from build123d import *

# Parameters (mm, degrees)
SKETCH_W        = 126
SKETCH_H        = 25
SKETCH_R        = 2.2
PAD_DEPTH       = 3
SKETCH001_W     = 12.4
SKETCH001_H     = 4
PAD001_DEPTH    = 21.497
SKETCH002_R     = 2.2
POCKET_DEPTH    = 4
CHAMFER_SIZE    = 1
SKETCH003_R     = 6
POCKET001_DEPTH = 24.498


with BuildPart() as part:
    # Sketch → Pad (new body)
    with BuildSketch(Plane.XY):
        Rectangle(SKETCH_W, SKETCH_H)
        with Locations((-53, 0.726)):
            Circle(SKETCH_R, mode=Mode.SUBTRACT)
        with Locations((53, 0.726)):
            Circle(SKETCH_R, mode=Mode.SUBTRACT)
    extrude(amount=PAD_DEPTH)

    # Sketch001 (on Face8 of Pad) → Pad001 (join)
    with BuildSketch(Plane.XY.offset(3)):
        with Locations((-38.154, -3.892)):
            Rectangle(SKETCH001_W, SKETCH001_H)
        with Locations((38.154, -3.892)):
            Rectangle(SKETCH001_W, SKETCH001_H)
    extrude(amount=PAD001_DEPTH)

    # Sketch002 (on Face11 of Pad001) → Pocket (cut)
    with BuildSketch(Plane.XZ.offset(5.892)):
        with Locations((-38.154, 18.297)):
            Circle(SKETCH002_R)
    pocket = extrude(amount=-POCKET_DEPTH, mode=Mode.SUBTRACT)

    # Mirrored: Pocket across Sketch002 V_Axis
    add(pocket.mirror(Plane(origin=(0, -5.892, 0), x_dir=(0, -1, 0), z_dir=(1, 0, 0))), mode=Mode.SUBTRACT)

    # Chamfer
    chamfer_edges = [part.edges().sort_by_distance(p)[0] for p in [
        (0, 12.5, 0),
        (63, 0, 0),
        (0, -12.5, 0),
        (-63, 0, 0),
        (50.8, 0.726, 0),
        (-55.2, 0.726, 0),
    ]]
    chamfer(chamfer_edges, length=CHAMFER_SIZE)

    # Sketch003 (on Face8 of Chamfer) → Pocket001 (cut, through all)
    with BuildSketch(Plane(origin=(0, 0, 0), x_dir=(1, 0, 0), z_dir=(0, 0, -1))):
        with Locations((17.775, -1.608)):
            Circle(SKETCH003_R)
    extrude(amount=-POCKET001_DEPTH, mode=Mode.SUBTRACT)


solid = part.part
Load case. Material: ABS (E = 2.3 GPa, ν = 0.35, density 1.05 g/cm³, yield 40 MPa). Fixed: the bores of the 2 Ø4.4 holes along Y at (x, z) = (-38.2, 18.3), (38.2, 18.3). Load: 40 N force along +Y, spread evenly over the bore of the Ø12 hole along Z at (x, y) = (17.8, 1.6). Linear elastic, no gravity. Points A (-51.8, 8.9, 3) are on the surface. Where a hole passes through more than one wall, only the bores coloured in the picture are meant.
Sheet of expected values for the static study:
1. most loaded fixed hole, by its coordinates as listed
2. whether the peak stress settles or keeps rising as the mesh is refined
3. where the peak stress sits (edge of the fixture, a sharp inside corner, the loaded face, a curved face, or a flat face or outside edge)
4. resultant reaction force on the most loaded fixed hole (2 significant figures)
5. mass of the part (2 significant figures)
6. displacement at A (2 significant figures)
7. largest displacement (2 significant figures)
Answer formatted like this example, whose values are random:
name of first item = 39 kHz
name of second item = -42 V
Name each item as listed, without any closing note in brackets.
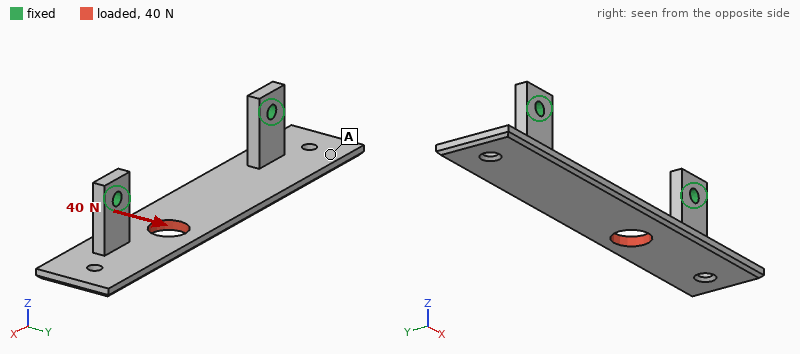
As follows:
most loaded fixed hole, by its coordinates as listed = (38.2, 18.3)
whether the peak stress settles or keeps rising as the mesh is refined = keeps rising
where the peak stress sits = edge of the fixture
resultant reaction force on the most loaded fixed hole = 29 N
mass of the part = 11 g
displacement at A = 0.15 mm
largest displacement = 0.42 mm
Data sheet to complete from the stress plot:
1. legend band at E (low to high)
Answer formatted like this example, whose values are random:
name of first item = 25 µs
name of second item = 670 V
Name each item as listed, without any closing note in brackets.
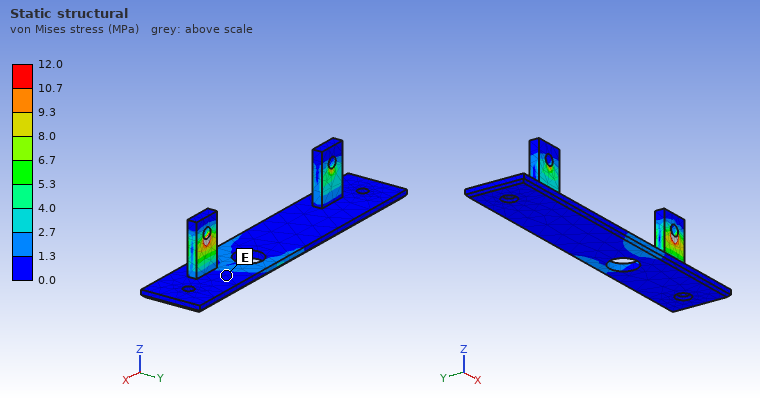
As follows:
legend band at E = 0.0 to 1.3 MPa
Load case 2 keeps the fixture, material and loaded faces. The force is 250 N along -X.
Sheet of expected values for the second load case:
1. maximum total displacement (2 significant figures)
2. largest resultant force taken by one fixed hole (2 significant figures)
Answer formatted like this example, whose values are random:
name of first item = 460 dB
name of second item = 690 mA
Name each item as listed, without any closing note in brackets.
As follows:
maximum total displacement = 0.61 mm
largest resultant force taken by one fixed hole = 130 N
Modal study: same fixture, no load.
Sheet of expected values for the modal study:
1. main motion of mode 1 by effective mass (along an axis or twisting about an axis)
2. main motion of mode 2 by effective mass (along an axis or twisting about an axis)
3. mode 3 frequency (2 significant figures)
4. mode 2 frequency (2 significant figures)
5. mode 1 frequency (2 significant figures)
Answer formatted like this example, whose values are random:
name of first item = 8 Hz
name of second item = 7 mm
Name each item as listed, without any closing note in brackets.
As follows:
main motion of mode 1 by effective mass = along Y
main motion of mode 2 by effective mass = twisting about Z
mode 3 frequency = 880 Hz
mode 2 frequency = 780 Hz
mode 1 frequency = 590 Hz
